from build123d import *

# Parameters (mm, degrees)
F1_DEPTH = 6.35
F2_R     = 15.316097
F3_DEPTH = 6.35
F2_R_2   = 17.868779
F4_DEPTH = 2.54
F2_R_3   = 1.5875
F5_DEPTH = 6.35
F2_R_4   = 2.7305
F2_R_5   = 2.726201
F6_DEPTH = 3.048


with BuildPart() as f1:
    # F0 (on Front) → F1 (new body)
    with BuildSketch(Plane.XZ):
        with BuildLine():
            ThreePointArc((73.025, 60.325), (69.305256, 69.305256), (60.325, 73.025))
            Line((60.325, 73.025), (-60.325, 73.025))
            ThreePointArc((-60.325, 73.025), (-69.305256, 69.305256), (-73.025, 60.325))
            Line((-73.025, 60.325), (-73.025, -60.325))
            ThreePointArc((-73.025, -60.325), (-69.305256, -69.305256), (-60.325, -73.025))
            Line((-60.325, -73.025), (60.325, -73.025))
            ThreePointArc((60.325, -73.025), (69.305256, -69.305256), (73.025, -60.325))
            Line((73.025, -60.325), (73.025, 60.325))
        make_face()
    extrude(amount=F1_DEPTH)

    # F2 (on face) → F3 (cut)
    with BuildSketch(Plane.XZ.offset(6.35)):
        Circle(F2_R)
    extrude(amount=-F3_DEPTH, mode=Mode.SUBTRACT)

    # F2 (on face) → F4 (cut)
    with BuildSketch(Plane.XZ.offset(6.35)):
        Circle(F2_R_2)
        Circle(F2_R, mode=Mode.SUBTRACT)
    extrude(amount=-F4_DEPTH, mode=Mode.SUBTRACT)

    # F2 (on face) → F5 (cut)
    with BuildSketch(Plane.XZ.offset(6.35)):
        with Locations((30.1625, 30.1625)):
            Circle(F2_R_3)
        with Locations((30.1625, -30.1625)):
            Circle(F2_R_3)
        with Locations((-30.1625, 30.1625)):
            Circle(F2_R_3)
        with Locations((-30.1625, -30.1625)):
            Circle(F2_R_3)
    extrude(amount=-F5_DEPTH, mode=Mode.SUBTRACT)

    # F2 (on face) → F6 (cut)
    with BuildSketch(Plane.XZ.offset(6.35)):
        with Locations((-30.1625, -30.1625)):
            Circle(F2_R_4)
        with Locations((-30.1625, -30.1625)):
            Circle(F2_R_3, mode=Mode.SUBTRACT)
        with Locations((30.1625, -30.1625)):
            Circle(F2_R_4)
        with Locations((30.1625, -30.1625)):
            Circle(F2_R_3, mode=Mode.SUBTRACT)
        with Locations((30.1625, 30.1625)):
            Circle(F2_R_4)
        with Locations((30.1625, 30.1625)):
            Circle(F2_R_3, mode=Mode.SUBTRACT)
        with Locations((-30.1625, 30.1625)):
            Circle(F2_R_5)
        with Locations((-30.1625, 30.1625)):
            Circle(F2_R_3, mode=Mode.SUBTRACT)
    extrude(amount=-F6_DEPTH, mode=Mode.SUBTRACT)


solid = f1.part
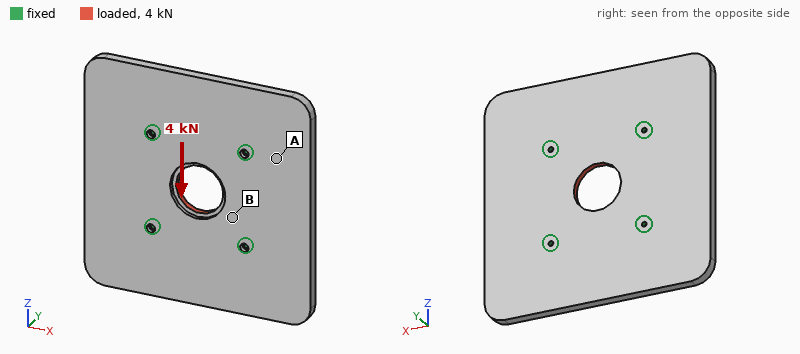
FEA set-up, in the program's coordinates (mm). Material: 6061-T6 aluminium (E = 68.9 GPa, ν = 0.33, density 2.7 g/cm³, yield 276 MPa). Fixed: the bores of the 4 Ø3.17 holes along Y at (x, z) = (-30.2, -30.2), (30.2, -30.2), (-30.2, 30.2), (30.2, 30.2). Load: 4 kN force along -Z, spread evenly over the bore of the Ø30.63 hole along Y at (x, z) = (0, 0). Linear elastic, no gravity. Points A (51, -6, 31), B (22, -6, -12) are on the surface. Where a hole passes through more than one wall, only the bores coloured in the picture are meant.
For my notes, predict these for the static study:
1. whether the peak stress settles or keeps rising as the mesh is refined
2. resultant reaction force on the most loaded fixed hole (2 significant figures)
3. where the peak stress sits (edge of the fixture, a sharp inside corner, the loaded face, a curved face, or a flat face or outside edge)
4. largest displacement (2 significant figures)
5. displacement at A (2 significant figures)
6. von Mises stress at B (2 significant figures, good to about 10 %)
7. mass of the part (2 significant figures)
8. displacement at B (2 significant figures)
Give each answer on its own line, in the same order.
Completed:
keeps rising
1.0 kN
edge of the fixture
6.5 µm
2.3 µm
5.0 MPa
350 g
2.9 µm
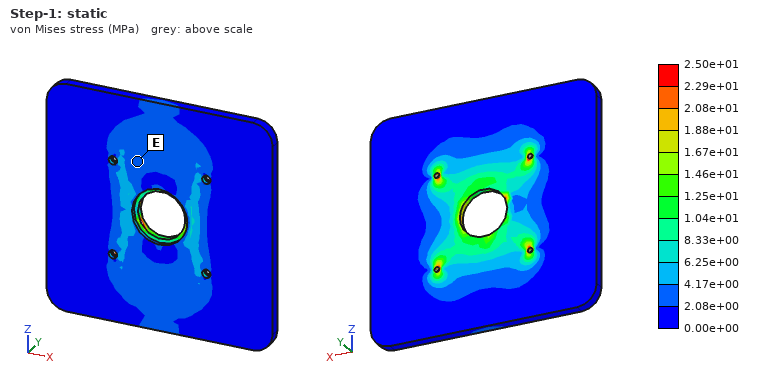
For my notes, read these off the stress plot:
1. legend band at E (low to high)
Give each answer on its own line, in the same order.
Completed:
2.08e+00 to 4.17e+00 MPa
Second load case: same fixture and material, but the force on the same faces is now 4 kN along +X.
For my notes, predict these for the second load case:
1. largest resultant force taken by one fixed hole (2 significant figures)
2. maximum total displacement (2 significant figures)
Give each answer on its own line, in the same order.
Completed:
1.0 kN
6.5 µm
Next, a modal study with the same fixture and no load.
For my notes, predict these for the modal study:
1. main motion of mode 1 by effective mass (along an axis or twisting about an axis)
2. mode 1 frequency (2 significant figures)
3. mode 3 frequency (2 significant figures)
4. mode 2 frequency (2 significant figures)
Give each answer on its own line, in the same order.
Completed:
along Y
1600 Hz
1800 Hz
1700 Hz
